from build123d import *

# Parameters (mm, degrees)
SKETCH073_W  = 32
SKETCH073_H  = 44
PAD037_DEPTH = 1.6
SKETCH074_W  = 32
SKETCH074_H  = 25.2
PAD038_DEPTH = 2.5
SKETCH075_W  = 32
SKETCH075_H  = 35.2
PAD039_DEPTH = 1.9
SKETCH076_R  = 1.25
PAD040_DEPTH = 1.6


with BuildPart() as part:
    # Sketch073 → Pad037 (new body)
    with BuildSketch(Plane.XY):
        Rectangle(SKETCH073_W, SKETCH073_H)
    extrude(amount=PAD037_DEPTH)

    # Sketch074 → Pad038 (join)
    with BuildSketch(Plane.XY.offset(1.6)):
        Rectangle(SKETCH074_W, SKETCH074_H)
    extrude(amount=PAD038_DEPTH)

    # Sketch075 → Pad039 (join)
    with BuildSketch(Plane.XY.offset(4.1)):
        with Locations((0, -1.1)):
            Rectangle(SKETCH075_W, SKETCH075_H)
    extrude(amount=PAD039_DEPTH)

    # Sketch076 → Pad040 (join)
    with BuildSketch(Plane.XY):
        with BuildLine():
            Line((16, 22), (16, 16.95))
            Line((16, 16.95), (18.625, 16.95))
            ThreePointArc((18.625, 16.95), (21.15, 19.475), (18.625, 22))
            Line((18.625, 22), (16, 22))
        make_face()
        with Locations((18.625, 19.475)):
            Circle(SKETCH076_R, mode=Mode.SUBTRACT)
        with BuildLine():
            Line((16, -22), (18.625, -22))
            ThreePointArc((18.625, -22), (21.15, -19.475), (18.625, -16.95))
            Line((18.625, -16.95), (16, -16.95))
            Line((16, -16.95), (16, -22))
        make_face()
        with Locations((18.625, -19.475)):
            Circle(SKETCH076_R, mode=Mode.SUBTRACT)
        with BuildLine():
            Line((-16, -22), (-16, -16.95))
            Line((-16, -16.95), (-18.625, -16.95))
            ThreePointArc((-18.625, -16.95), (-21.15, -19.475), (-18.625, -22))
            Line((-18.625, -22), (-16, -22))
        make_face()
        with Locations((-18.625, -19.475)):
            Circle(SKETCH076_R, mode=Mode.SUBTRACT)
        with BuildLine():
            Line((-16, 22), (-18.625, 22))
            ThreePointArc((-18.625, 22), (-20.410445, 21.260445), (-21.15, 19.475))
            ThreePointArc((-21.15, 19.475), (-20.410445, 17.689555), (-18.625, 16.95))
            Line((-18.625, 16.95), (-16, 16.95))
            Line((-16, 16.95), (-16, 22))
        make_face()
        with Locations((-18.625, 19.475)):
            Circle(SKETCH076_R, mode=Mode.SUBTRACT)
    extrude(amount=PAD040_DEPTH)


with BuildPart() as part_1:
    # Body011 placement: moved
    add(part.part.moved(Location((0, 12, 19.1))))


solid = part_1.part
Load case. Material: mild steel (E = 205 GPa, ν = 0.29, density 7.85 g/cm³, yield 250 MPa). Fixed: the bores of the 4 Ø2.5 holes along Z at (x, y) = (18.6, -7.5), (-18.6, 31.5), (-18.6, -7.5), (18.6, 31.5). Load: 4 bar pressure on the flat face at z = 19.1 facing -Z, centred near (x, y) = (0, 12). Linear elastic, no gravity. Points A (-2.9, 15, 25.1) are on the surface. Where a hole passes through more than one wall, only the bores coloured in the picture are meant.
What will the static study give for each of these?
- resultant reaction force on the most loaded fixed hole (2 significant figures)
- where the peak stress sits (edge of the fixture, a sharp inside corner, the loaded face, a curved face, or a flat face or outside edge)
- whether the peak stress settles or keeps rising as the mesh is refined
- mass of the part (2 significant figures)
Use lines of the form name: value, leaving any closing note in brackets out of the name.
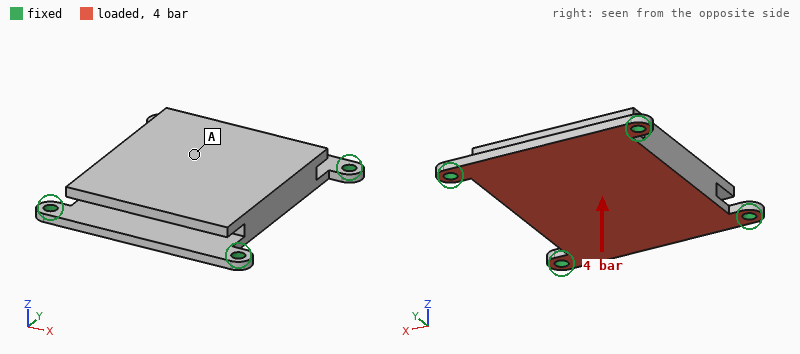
resultant reaction force on the most loaded fixed hole: 160 N
where the peak stress sits: edge of the fixture
whether the peak stress settles or keeps rising as the mesh is refined: keeps rising
mass of the part: 51 g
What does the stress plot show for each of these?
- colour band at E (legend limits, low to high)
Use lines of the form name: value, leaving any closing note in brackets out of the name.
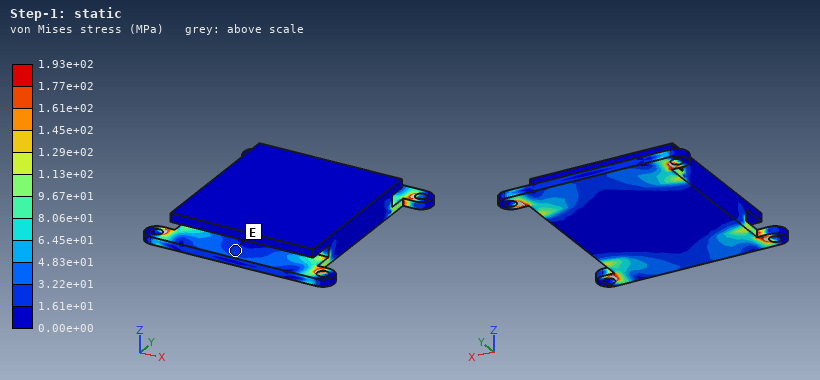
colour band at E: 1.61e+01 to 3.22e+01 MPa
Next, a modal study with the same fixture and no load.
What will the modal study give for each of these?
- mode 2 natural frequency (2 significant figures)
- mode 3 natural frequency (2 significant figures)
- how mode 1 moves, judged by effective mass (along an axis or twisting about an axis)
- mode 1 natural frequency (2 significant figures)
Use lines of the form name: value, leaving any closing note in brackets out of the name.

mode 2 natural frequency: 5800 Hz
mode 3 natural frequency: 6200 Hz
how mode 1 moves, judged by effective mass: along Z
mode 1 natural frequency: 3600 Hz
